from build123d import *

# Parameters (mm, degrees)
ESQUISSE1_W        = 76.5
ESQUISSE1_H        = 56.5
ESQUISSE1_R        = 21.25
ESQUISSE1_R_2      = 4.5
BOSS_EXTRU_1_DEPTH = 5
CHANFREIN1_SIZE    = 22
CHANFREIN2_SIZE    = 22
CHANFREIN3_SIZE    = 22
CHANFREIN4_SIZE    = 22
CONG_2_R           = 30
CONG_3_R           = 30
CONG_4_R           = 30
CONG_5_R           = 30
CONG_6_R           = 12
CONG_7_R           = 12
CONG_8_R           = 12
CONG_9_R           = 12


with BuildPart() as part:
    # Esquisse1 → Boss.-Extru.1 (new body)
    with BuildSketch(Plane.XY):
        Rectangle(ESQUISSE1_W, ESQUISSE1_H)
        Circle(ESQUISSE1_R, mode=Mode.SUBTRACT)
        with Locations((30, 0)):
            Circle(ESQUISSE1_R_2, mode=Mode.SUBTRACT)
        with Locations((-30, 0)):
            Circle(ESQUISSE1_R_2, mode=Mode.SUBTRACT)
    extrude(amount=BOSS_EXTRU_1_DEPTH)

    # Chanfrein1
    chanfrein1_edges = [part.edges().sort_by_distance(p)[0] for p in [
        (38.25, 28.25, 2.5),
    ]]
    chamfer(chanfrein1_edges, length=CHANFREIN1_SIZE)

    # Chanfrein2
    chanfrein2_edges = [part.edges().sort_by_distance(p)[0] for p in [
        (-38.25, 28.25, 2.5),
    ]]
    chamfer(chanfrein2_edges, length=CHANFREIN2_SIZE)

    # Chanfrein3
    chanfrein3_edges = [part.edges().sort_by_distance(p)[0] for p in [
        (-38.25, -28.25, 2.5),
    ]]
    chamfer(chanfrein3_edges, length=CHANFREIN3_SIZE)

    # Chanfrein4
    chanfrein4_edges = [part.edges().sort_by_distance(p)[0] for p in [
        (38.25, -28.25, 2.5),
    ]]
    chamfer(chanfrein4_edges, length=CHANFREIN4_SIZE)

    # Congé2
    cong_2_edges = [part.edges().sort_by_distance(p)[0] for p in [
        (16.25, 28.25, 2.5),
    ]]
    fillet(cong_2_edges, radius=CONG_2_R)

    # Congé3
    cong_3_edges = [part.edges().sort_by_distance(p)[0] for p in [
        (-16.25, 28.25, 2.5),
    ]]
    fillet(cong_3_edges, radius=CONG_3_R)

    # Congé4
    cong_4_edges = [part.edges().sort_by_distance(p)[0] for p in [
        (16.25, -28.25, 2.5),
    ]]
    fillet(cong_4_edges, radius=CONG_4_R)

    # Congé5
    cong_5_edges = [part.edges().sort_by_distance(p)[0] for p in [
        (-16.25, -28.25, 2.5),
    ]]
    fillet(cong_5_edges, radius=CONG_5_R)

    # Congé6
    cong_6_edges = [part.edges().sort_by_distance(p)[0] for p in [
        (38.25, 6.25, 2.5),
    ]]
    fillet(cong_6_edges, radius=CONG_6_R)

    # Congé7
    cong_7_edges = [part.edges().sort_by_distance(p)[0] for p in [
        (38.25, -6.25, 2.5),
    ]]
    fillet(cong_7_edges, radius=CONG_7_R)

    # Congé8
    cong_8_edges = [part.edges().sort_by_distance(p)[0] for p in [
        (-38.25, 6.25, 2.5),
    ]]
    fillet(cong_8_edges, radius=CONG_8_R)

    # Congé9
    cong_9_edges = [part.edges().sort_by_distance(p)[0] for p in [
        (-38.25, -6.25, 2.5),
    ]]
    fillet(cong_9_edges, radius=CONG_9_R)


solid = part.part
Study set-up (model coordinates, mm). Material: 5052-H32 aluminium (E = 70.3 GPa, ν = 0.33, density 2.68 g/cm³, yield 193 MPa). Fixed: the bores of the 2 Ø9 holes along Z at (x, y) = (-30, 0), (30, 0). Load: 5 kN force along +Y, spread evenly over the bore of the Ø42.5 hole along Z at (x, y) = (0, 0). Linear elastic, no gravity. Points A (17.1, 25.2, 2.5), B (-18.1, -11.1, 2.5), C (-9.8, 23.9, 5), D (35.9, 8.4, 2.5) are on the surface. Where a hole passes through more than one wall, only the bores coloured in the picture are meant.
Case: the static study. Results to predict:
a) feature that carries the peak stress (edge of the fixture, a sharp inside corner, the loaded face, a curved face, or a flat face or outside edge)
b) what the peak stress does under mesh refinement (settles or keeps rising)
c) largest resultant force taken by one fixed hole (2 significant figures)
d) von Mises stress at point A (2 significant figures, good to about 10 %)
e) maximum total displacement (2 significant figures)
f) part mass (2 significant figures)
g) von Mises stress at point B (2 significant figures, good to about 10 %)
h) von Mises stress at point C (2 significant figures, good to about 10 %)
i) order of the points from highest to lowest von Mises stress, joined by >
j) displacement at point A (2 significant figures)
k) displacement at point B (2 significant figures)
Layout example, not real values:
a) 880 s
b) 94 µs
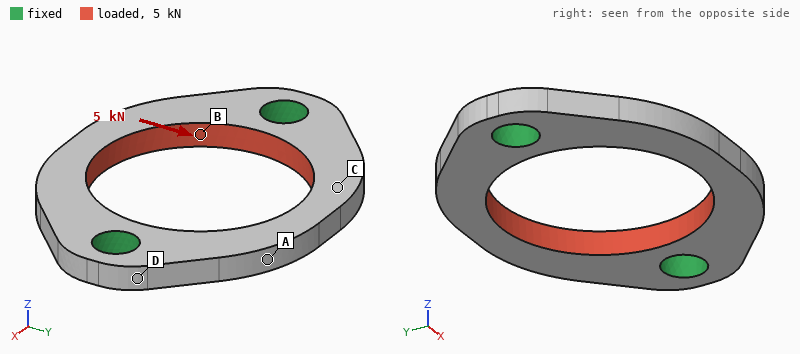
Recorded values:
a) edge of the fixture
b) keeps rising
c) 2.5 kN
d) 12 MPa
e) 21 µm
f) 23 g
g) 42 MPa
h) 23 MPa
i) B > C > A > D
j) 10 µm
k) 7.0 µm
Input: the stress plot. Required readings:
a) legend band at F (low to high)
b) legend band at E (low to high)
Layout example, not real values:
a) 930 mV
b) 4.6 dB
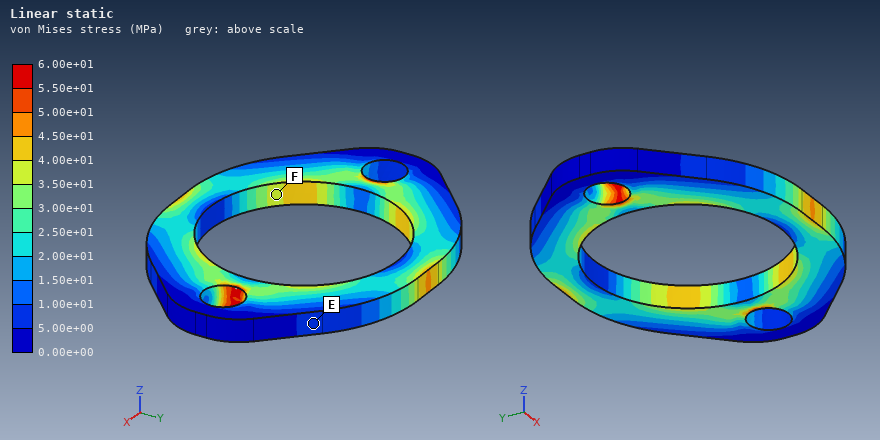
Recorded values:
a) 3.50e+01 to 4.00e+01 MPa
b) 5.00e+00 to 1.00e+01 MPa
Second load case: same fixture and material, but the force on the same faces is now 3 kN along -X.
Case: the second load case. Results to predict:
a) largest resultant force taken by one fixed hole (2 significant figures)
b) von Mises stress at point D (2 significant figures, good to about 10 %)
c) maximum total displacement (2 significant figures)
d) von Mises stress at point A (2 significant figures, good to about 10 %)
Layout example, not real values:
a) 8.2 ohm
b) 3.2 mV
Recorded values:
a) 1.5 kN
b) 16 MPa
c) 14 µm
d) 13 MPa
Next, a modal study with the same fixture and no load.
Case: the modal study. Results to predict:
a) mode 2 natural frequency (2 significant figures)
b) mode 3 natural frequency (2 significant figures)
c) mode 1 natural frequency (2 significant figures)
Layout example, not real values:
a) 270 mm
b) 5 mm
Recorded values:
a) 4500 Hz
b) 11 kHz
c) 4400 Hz
